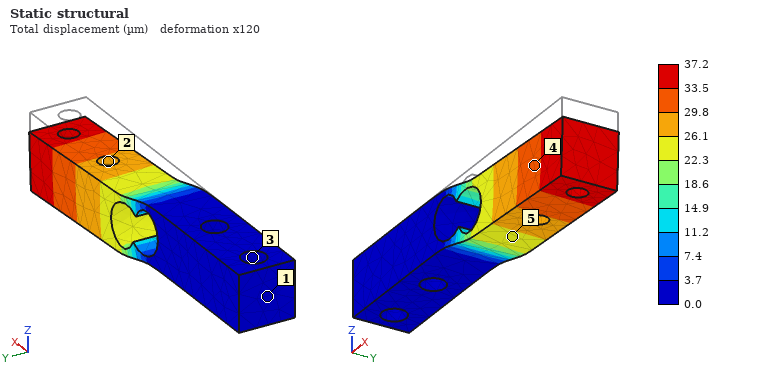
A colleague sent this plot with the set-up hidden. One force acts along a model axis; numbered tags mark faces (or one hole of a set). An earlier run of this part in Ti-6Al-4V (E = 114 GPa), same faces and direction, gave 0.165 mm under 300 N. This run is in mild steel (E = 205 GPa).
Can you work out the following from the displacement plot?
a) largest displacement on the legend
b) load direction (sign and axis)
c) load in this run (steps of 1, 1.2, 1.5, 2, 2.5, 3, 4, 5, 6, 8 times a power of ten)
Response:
37.2 µm
-Z
120 N
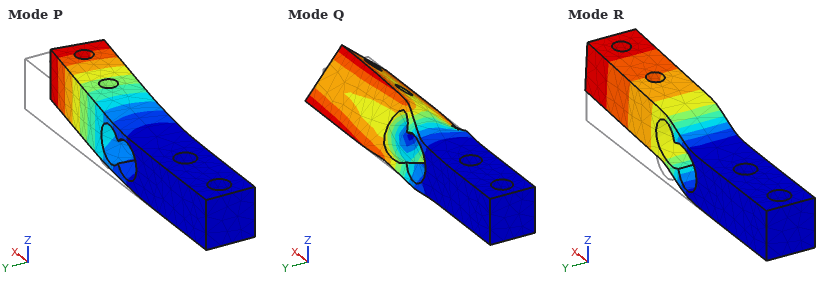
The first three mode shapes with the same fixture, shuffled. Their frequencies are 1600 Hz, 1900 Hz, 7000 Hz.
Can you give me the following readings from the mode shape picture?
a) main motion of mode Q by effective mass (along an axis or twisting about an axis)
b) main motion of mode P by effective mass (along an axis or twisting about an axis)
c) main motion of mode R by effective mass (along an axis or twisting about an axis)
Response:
twisting about X
along Y
along Z
